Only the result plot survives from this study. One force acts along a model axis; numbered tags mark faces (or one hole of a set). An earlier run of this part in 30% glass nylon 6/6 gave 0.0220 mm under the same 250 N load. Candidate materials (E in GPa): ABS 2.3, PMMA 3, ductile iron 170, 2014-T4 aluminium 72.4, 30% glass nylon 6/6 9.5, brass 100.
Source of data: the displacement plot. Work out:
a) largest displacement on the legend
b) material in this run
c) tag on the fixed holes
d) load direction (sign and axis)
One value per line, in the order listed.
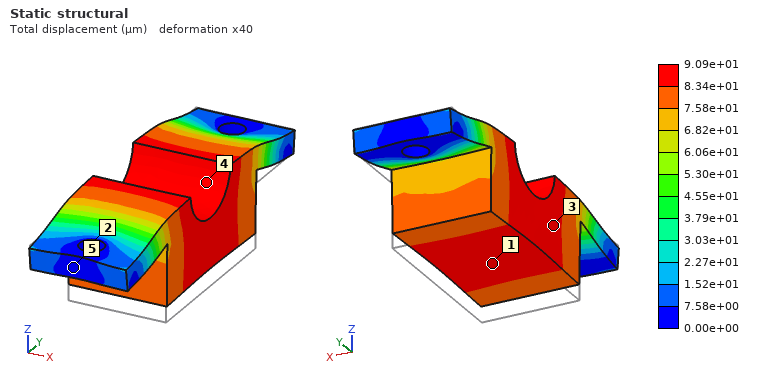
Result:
9.09e+01 µm
ABS
2
+Z
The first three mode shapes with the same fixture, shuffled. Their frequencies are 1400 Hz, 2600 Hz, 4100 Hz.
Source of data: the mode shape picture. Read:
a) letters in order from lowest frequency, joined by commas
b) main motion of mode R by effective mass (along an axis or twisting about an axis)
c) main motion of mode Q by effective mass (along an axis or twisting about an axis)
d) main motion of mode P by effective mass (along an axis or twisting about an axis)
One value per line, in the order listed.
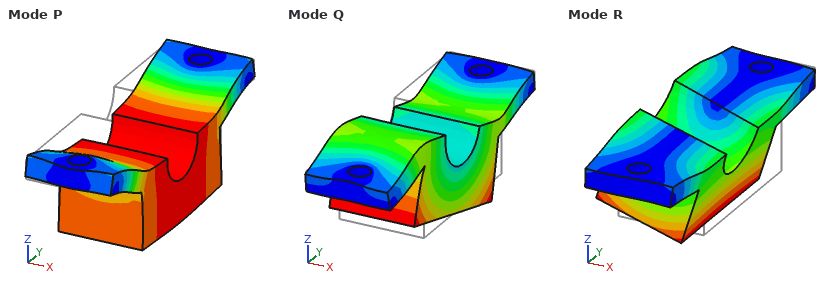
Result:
R, P, Q
along X
along Y
along Z
